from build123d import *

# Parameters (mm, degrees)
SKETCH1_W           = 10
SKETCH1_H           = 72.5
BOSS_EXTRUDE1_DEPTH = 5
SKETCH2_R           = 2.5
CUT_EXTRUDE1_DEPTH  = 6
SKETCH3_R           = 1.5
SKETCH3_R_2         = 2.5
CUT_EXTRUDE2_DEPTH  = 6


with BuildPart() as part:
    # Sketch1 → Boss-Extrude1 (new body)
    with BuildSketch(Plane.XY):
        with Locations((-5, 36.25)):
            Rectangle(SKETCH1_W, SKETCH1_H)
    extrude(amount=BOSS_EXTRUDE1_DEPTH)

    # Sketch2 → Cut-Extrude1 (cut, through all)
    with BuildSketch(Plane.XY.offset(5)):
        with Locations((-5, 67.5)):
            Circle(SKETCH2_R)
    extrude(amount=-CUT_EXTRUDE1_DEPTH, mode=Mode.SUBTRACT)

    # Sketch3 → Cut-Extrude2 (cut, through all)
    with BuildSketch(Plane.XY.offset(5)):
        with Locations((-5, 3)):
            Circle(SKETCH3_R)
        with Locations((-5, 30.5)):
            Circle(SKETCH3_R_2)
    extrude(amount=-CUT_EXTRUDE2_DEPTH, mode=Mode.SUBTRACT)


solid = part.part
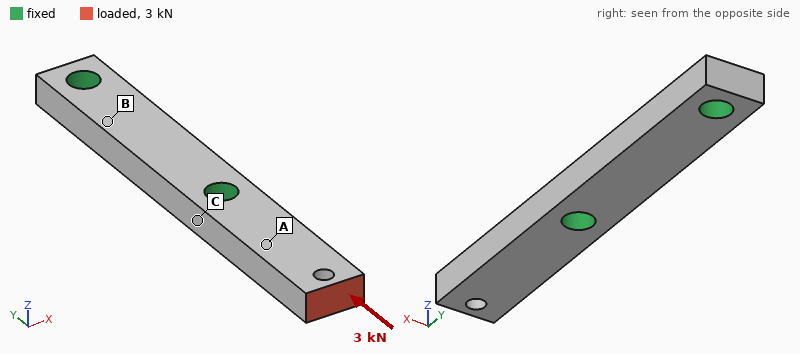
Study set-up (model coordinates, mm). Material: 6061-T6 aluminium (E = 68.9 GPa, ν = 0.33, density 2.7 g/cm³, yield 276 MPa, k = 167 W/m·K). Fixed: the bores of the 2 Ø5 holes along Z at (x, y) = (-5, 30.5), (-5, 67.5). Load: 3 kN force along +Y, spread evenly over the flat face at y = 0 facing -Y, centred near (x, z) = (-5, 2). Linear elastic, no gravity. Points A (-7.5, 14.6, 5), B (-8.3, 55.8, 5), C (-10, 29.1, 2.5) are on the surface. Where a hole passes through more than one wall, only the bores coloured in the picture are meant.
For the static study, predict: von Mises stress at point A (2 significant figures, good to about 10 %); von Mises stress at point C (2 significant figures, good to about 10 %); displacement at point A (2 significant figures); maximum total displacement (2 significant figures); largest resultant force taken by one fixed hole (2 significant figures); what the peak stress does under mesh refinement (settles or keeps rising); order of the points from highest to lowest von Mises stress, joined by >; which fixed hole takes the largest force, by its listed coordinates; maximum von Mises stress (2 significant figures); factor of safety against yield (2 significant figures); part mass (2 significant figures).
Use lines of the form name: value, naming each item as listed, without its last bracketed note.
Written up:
von Mises stress at point A: 60 MPa
von Mises stress at point C: 32 MPa
displacement at point A: 13 µm
maximum total displacement: 32 µm
largest resultant force taken by one fixed hole: 3.0 kN
what the peak stress does under mesh refinement: settles
order of the points from highest to lowest von Mises stress, joined by >: A > C > B
which fixed hole takes the largest force, by its listed coordinates: (-5, 30.5)
maximum von Mises stress: 240 MPa
factor of safety against yield: 1.2
part mass: 9.2 g
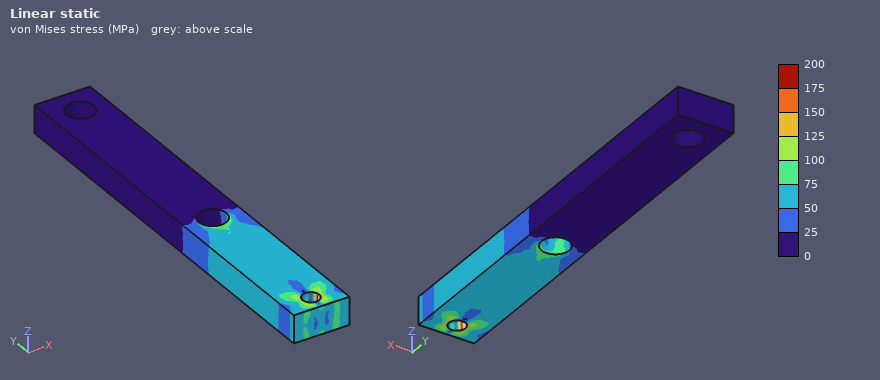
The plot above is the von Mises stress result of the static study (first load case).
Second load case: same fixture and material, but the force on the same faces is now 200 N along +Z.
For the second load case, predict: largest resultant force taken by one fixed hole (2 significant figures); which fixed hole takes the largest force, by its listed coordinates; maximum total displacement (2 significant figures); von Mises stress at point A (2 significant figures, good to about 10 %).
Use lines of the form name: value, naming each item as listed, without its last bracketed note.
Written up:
largest resultant force taken by one fixed hole: 200 N
which fixed hole takes the largest force, by its listed coordinates: (-5, 30.5)
maximum total displacement: 0.23 mm
von Mises stress at point A: 70 MPa
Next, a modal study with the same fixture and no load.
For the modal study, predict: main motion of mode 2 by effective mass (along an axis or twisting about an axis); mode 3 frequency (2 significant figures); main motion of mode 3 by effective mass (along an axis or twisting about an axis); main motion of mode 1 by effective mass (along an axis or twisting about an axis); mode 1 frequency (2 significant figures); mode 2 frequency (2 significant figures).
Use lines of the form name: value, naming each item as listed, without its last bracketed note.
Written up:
main motion of mode 2 by effective mass: along X
mode 3 frequency: 20 kHz
main motion of mode 3 by effective mass: along Z
main motion of mode 1 by effective mass: along Z
mode 1 frequency: 5000 Hz
mode 2 frequency: 8200 Hz
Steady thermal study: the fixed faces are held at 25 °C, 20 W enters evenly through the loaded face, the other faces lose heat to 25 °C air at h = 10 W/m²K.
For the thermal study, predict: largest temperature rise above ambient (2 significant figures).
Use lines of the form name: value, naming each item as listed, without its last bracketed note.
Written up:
largest temperature rise above ambient: 74 K
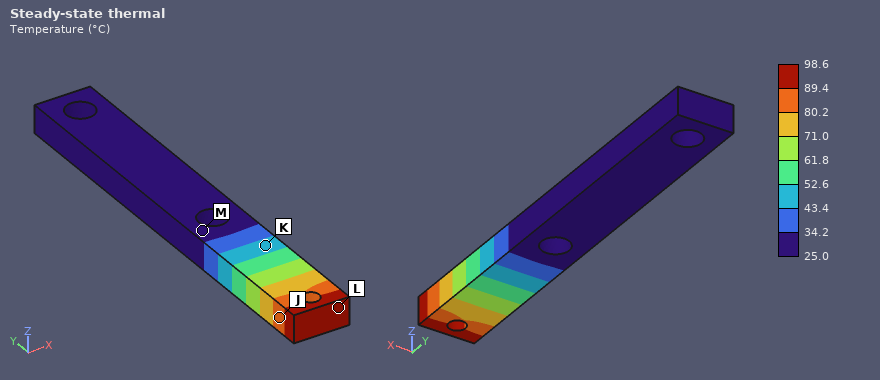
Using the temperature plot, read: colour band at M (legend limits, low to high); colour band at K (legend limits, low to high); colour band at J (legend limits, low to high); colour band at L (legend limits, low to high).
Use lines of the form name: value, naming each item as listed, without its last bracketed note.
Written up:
colour band at M: 25.0 to 34.2 °C
colour band at K: 43.4 to 52.6 °C
colour band at J: 80.2 to 89.4 °C
colour band at L: 89.4 to 98.6 °C
